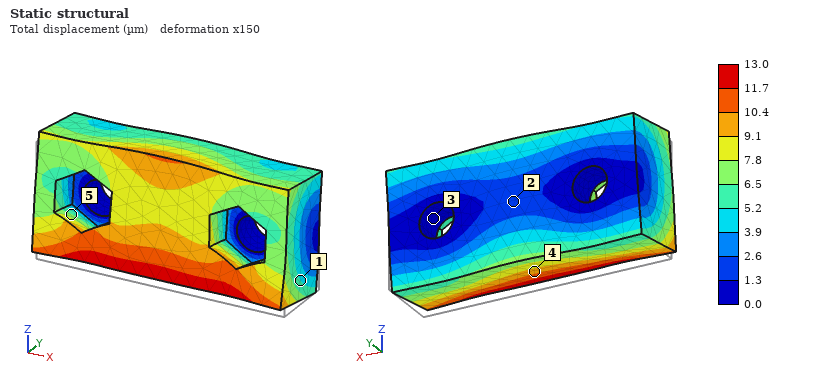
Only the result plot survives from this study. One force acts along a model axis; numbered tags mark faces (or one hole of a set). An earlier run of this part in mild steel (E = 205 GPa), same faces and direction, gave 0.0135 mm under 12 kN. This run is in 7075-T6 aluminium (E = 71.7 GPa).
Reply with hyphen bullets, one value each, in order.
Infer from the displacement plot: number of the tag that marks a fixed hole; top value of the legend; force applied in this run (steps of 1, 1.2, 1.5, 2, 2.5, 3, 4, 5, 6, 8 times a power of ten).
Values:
- 3
- 13.0 µm
- 4 kN
